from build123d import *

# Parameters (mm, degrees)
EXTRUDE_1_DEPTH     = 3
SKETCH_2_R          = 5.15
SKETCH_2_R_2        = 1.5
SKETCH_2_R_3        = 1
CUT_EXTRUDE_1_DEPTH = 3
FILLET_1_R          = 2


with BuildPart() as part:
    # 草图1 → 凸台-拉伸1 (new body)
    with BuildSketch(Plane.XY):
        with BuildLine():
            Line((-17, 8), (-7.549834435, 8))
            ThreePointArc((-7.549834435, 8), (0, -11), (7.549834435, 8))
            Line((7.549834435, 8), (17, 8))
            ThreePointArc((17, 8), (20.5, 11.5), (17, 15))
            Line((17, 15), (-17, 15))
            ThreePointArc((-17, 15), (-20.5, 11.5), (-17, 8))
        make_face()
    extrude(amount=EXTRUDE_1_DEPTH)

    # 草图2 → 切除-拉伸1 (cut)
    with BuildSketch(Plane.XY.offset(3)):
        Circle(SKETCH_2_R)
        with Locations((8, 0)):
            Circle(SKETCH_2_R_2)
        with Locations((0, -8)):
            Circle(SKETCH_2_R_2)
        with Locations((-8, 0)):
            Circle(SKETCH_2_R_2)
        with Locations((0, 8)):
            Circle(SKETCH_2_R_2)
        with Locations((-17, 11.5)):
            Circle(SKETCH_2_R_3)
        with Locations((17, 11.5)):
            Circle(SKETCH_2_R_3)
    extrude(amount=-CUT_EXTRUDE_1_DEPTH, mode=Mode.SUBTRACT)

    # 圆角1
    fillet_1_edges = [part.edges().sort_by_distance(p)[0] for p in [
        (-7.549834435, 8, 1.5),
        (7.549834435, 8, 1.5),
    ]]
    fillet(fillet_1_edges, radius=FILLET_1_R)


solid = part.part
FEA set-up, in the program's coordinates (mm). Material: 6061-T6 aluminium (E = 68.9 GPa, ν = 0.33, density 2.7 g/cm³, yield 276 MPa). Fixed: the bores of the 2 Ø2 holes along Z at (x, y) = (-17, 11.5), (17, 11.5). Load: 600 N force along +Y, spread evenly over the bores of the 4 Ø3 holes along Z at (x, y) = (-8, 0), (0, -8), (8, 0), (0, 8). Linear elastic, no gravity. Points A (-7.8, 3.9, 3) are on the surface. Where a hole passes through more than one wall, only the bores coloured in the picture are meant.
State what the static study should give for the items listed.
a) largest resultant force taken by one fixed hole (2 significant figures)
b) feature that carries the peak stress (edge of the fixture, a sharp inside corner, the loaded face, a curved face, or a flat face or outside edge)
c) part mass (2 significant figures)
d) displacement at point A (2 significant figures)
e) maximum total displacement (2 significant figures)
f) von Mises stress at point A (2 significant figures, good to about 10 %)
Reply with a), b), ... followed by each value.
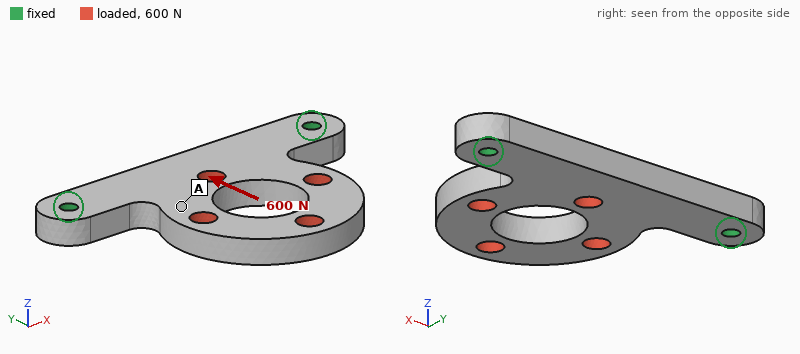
a) 320 N
b) edge of the fixture
c) 4.2 g
d) 15 µm
e) 18 µm
f) 20 MPa
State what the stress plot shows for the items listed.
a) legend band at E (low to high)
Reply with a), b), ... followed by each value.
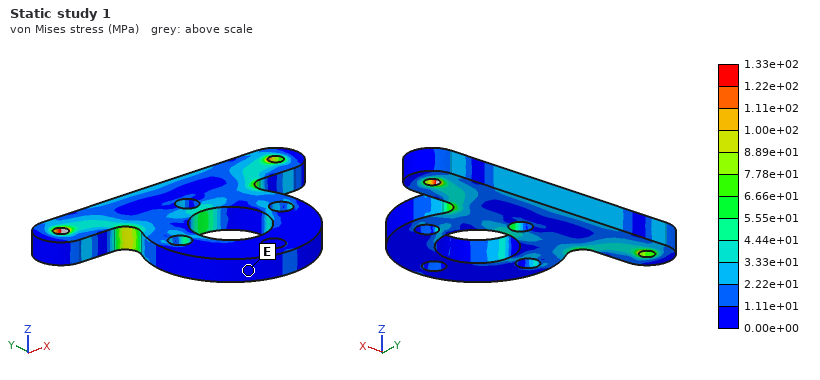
a) 0.00e+00 to 1.11e+01 MPa
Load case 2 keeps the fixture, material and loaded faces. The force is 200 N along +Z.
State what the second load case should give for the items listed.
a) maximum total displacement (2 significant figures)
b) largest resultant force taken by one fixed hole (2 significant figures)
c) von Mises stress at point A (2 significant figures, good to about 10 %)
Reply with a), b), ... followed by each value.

a) 0.32 mm
b) 100 N
c) 53 MPa
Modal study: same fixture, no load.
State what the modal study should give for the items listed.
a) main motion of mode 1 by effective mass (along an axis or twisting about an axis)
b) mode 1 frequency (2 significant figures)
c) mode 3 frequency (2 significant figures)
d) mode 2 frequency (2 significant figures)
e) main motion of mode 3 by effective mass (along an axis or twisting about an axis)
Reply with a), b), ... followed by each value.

a) along Z
b) 3400 Hz
c) 12 kHz
d) 11 kHz
e) along Z
